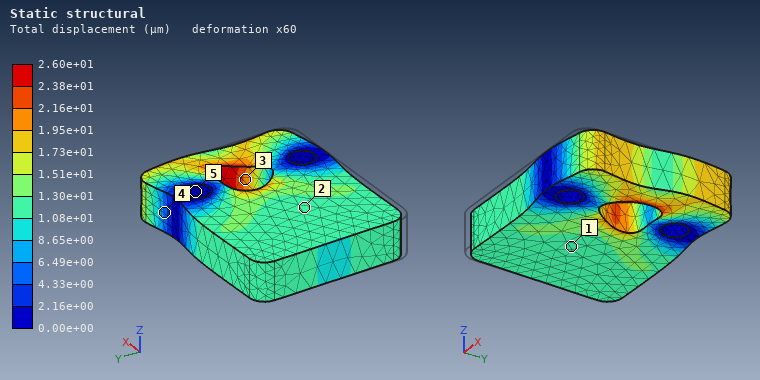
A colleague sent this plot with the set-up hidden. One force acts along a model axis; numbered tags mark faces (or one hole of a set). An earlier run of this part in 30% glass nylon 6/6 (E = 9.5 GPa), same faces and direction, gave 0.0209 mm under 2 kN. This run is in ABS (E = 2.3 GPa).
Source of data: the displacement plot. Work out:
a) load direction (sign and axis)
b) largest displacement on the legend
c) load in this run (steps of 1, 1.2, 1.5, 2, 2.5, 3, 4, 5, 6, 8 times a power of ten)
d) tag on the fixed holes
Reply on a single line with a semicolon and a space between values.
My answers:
+Y; 2.60e+01 µm; 600 N; 5
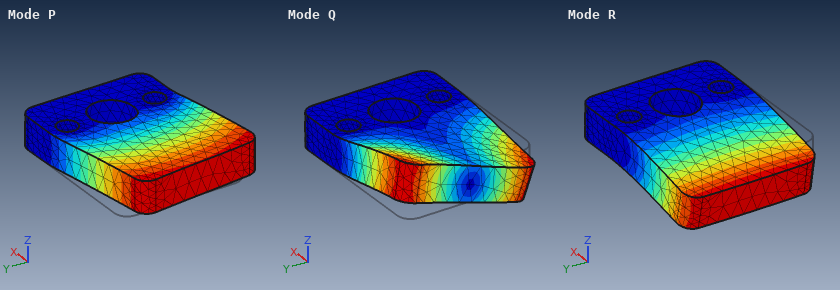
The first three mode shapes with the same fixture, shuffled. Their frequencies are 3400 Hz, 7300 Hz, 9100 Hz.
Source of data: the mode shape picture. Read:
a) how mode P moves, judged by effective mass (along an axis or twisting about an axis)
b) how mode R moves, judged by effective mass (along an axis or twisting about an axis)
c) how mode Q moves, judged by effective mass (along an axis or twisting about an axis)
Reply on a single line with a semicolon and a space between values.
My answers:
along Y; along Z; twisting about X
